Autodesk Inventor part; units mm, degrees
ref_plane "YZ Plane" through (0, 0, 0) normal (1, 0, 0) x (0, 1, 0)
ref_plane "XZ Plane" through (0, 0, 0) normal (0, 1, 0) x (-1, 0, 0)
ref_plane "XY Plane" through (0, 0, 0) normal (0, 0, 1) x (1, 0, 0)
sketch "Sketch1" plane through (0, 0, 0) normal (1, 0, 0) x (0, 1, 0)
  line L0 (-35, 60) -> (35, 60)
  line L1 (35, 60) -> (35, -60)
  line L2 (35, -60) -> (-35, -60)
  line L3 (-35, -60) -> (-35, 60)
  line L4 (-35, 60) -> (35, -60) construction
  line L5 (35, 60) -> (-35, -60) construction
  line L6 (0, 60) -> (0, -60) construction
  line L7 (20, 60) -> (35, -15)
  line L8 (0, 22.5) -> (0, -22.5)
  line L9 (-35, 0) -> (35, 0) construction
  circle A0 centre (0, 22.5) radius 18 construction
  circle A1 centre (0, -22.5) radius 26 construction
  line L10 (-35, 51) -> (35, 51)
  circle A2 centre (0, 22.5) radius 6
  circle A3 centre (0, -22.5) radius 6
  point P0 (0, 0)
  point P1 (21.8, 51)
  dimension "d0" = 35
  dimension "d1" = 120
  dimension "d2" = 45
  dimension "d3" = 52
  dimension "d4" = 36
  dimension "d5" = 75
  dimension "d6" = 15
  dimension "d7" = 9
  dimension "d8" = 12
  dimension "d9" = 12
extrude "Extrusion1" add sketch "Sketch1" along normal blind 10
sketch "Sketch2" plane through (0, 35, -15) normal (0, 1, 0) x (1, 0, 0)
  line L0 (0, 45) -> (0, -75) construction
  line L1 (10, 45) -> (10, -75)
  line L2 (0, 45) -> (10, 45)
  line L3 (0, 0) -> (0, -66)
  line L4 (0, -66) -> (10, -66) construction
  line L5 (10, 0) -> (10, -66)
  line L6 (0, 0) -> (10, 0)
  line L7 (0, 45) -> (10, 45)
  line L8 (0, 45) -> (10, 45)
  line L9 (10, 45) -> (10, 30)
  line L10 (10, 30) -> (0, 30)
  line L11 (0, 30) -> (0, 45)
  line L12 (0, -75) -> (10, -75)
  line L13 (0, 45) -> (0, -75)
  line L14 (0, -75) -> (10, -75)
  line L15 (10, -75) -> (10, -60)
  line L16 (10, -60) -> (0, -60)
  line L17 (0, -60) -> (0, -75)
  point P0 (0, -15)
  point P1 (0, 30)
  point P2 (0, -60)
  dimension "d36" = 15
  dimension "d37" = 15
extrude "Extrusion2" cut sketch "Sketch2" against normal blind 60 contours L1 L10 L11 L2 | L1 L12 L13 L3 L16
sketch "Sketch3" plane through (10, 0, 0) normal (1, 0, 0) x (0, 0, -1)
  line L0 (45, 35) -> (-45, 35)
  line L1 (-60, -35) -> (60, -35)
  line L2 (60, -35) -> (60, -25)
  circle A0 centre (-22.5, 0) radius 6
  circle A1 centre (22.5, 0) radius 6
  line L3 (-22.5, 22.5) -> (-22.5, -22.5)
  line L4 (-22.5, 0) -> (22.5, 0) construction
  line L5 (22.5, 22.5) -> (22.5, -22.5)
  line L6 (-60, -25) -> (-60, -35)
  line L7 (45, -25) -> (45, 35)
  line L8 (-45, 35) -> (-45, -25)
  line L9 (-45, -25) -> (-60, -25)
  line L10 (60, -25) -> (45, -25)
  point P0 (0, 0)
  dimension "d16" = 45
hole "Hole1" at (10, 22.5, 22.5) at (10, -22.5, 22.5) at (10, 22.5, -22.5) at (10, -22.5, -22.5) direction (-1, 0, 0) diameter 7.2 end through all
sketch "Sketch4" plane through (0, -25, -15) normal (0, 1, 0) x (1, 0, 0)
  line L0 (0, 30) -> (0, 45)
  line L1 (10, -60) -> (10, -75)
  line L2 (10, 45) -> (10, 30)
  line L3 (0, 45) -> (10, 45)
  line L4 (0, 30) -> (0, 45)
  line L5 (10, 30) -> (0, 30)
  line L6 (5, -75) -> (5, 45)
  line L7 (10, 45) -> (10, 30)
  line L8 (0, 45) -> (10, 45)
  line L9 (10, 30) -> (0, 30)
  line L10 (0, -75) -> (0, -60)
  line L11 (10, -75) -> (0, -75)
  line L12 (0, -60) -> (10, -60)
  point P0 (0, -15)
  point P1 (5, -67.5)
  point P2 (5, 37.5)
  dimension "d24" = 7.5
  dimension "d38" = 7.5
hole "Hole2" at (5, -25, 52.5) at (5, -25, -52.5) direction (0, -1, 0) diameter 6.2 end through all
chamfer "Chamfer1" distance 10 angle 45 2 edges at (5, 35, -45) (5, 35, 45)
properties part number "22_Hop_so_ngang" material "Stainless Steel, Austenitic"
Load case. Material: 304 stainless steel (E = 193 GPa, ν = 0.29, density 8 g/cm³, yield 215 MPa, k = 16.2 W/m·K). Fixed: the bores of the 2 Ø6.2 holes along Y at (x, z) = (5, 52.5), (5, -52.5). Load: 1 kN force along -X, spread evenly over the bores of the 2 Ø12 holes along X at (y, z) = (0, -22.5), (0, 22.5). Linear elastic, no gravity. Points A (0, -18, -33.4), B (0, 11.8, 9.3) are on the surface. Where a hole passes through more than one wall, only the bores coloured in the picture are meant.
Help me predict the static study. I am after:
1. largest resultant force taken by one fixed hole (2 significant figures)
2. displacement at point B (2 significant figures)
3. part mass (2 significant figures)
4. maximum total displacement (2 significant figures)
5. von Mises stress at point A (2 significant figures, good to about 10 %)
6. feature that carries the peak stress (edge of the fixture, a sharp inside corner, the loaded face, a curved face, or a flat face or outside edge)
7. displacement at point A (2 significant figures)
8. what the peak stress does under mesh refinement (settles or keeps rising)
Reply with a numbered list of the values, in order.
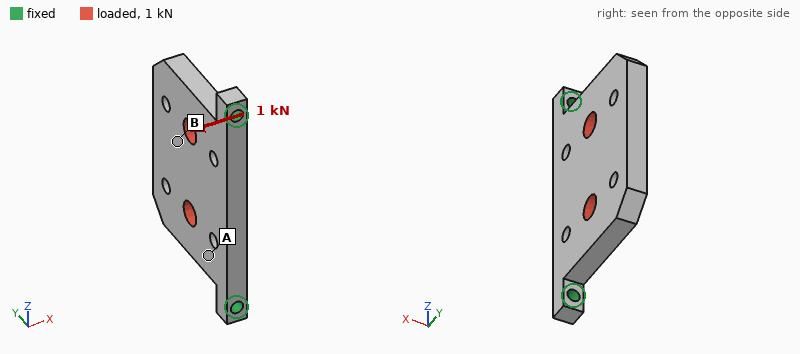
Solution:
1. 500 N
2. 0.079 mm
3. 480 g
4. 0.12 mm
5. 22 MPa
6. edge of the fixture
7. 0.023 mm
8. keeps rising
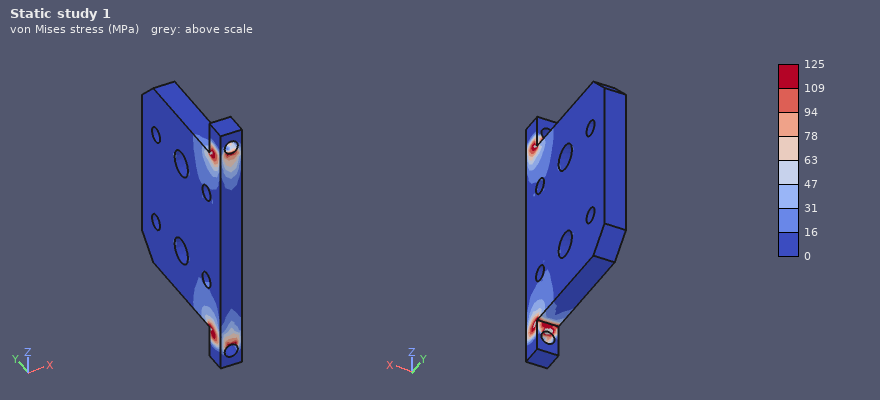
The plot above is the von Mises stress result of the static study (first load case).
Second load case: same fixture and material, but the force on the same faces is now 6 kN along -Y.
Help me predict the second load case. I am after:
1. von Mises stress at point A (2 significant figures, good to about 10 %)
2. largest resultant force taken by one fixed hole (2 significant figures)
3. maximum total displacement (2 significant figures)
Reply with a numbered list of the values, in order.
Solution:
1. 18 MPa
2. 3.4 kN
3. 10.0 µm
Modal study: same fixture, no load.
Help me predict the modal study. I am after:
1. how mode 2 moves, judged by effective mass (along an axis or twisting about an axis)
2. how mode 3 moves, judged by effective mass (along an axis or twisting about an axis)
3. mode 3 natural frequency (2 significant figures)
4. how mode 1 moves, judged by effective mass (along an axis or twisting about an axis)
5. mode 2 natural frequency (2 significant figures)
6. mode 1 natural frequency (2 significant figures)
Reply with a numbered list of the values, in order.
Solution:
1. twisting about Y
2. along X
3. 4000 Hz
4. along X
5. 2900 Hz
6. 820 Hz
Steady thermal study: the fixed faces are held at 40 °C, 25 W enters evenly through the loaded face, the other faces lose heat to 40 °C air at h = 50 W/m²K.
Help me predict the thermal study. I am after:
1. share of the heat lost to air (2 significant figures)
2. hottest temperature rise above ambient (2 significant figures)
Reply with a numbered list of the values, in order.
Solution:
1. 82 %
2. 44 K
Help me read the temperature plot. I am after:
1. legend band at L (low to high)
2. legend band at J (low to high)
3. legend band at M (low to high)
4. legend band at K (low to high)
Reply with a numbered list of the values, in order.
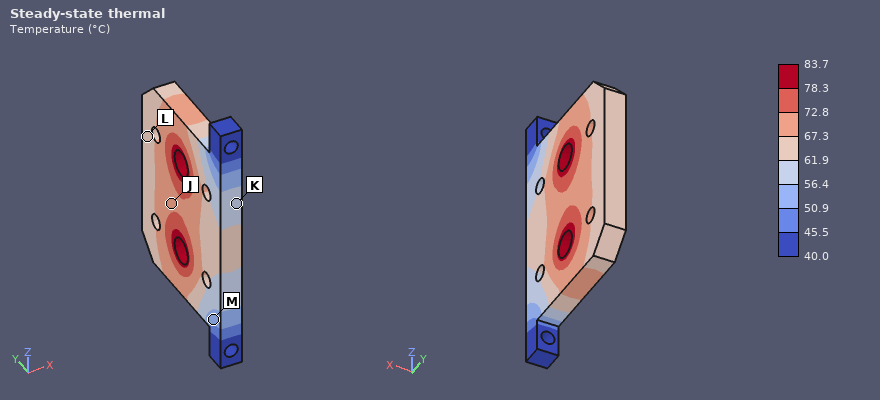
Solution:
1. 61.9 to 67.3 °C
2. 67.3 to 72.8 °C
3. 50.9 to 56.4 °C
4. 56.4 to 61.9 °C
